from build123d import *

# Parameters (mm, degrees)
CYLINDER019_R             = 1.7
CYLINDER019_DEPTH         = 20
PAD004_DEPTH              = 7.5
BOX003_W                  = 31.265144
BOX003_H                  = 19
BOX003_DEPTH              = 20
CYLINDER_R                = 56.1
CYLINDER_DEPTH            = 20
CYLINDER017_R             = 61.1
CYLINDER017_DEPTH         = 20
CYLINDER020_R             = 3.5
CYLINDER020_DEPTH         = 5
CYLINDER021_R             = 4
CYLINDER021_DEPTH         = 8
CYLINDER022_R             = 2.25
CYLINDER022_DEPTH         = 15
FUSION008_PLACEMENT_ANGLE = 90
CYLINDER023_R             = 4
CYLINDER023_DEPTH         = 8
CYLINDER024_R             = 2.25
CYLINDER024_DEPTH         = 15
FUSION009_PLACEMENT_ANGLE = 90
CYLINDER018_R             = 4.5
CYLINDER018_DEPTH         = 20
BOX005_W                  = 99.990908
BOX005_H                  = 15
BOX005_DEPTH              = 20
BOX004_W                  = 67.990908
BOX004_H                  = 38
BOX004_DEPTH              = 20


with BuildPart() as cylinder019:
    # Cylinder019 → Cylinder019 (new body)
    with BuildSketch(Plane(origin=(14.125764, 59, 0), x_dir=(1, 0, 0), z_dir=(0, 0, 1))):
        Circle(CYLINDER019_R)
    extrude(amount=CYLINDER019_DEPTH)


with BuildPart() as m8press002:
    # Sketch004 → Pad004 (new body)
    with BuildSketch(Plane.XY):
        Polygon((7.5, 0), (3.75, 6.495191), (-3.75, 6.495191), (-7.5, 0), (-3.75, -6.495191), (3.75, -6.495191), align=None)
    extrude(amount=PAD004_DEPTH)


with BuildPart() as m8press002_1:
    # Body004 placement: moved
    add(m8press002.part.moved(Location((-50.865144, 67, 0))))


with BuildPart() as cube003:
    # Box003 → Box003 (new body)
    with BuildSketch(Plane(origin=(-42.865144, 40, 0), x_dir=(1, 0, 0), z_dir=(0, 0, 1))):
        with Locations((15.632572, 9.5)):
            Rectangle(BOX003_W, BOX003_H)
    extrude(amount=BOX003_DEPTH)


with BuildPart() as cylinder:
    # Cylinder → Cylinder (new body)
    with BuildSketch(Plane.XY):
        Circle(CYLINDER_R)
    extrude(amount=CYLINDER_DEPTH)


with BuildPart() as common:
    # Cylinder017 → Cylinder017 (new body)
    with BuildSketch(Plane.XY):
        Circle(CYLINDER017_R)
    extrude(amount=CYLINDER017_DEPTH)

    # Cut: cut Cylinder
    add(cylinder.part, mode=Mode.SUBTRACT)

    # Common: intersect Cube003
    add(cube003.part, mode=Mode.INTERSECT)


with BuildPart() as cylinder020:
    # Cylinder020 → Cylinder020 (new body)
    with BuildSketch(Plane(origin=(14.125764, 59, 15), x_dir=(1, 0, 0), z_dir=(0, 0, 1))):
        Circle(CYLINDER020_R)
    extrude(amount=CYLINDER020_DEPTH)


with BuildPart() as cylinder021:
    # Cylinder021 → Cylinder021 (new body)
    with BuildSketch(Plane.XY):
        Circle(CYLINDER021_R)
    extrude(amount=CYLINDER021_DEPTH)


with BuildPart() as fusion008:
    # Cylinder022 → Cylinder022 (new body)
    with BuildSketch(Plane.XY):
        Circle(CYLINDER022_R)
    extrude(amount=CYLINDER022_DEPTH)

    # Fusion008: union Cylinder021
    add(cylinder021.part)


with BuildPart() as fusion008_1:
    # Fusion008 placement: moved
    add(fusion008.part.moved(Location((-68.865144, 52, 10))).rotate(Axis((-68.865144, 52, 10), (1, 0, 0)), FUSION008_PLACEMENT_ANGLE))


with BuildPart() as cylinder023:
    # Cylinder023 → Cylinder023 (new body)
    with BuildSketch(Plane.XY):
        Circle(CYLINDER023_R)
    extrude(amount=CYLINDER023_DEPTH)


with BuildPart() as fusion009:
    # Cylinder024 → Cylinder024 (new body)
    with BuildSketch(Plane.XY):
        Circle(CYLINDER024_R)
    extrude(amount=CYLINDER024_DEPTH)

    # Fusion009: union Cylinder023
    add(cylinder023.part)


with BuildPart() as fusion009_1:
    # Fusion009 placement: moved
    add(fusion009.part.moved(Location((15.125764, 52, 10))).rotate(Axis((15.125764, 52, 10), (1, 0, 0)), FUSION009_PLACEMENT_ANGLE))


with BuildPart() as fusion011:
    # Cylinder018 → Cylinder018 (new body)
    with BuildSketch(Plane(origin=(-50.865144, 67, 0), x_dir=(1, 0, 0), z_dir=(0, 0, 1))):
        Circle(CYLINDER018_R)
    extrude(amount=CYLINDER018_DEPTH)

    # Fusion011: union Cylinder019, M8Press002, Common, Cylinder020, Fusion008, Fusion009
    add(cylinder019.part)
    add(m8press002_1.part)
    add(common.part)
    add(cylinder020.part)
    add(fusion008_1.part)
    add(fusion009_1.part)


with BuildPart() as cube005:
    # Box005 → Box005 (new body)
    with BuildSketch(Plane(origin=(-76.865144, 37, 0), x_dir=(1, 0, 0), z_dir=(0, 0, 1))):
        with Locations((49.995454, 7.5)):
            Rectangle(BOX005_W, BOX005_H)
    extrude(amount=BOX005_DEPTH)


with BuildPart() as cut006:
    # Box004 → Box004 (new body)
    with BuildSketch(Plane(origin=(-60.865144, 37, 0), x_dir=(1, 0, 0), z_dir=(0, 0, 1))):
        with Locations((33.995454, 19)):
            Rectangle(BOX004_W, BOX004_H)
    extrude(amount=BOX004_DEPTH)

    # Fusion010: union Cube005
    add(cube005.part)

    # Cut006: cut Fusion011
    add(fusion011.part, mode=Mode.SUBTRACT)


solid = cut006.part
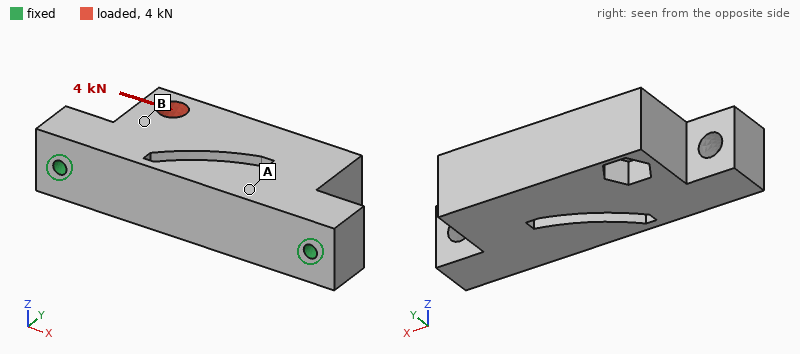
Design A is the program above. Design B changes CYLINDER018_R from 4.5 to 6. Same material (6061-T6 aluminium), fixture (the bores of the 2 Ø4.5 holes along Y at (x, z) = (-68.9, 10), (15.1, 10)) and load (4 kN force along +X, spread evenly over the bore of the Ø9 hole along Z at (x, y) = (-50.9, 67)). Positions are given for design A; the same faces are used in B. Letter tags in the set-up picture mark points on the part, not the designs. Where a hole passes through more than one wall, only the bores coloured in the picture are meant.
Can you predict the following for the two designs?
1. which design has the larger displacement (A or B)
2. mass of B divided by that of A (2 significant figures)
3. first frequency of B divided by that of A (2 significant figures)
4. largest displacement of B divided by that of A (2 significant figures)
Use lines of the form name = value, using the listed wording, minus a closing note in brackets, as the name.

which design has the larger displacement = B
mass of B divided by that of A = 0.99
first frequency of B divided by that of A = 1.0
largest displacement of B divided by that of A = 1.2
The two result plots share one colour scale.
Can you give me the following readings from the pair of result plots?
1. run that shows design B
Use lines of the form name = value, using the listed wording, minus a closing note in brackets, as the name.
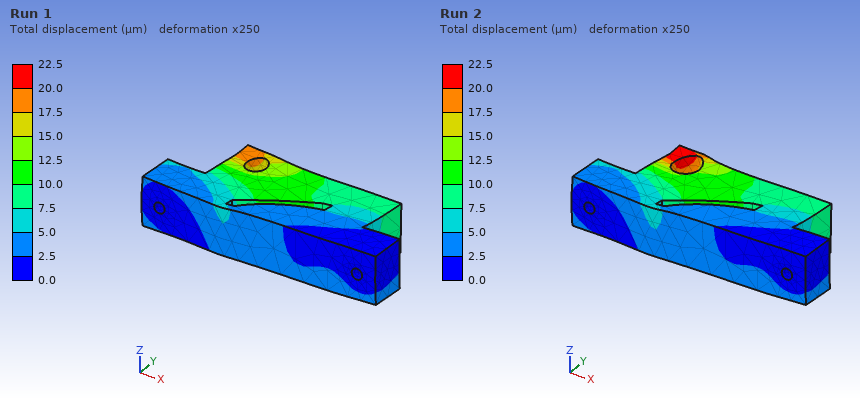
run that shows design B = Run 2
